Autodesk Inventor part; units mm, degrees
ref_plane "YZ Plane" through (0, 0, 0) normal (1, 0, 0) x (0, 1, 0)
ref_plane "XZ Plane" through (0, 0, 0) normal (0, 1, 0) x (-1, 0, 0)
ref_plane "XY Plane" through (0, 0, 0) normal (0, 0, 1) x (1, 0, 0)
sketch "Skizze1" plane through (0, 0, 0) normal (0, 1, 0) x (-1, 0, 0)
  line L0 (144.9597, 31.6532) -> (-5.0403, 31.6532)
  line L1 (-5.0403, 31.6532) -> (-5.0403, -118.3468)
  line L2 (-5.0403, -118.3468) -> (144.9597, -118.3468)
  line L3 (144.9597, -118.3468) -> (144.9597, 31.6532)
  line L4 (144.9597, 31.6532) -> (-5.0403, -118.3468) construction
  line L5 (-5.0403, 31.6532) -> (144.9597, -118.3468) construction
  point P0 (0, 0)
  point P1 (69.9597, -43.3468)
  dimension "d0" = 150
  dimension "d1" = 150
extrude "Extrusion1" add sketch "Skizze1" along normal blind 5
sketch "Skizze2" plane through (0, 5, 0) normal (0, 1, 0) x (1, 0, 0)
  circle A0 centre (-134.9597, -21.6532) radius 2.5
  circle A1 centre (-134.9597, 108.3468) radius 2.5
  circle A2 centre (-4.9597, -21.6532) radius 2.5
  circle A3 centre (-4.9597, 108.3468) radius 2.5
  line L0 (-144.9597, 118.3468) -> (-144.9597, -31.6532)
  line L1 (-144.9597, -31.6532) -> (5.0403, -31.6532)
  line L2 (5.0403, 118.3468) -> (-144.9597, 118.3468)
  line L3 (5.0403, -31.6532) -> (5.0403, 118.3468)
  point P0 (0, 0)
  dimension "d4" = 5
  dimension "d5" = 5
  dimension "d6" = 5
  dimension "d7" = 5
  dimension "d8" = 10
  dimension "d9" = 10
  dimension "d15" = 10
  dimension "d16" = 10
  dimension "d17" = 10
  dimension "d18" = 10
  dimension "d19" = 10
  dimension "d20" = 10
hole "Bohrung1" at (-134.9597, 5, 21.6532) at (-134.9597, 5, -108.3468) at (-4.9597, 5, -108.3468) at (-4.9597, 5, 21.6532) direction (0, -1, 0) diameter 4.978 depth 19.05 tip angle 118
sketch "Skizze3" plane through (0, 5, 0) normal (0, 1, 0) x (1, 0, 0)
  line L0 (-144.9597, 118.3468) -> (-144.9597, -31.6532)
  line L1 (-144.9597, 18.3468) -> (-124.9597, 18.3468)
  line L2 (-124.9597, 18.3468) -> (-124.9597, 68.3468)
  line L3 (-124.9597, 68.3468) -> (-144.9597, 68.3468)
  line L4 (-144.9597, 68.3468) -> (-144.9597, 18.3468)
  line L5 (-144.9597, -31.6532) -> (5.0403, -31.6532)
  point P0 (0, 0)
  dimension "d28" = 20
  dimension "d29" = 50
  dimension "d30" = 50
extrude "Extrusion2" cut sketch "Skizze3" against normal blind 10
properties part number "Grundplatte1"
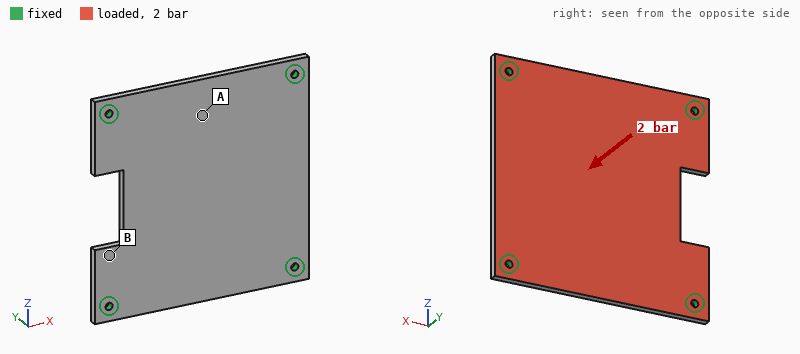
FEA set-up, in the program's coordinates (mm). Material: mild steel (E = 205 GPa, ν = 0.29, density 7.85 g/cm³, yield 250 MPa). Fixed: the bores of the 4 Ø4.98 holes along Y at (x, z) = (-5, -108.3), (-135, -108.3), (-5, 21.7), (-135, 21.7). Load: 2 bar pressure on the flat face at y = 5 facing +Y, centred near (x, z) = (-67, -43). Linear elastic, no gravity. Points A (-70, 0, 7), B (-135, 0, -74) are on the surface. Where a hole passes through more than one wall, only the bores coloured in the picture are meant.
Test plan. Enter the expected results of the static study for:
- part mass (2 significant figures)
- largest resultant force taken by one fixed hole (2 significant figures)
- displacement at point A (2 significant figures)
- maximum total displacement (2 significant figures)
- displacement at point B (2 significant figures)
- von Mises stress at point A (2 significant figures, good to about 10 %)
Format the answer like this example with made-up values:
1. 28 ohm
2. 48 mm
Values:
1. 840 g
2. 1.1 kN
3. 0.14 mm
4. 0.21 mm
5. 0.072 mm
6. 45 MPa
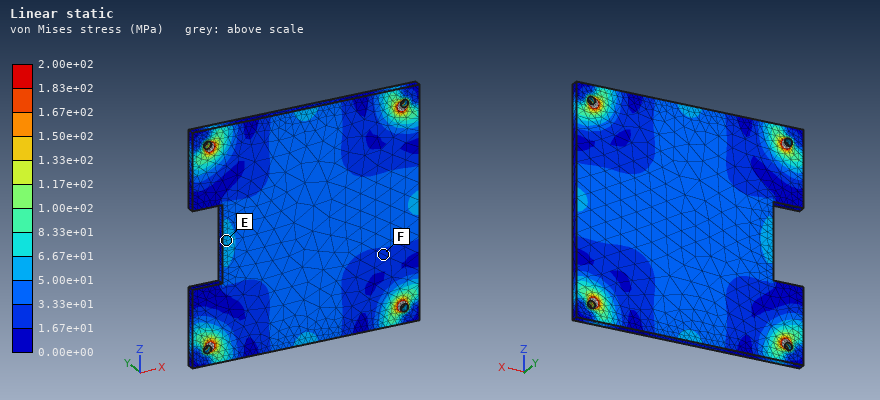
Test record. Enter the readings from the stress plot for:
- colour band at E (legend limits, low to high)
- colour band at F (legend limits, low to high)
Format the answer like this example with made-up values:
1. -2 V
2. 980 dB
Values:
1. 5.00e+01 to 6.67e+01 MPa
2. 1.67e+01 to 3.33e+01 MPa
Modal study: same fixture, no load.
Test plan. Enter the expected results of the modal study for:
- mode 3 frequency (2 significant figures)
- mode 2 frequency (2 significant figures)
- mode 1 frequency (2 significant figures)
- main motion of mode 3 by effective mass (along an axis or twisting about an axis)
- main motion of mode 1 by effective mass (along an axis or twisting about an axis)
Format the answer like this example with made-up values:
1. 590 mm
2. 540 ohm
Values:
1. 1700 Hz
2. 1600 Hz
3. 940 Hz
4. twisting about Z
5. along Y
